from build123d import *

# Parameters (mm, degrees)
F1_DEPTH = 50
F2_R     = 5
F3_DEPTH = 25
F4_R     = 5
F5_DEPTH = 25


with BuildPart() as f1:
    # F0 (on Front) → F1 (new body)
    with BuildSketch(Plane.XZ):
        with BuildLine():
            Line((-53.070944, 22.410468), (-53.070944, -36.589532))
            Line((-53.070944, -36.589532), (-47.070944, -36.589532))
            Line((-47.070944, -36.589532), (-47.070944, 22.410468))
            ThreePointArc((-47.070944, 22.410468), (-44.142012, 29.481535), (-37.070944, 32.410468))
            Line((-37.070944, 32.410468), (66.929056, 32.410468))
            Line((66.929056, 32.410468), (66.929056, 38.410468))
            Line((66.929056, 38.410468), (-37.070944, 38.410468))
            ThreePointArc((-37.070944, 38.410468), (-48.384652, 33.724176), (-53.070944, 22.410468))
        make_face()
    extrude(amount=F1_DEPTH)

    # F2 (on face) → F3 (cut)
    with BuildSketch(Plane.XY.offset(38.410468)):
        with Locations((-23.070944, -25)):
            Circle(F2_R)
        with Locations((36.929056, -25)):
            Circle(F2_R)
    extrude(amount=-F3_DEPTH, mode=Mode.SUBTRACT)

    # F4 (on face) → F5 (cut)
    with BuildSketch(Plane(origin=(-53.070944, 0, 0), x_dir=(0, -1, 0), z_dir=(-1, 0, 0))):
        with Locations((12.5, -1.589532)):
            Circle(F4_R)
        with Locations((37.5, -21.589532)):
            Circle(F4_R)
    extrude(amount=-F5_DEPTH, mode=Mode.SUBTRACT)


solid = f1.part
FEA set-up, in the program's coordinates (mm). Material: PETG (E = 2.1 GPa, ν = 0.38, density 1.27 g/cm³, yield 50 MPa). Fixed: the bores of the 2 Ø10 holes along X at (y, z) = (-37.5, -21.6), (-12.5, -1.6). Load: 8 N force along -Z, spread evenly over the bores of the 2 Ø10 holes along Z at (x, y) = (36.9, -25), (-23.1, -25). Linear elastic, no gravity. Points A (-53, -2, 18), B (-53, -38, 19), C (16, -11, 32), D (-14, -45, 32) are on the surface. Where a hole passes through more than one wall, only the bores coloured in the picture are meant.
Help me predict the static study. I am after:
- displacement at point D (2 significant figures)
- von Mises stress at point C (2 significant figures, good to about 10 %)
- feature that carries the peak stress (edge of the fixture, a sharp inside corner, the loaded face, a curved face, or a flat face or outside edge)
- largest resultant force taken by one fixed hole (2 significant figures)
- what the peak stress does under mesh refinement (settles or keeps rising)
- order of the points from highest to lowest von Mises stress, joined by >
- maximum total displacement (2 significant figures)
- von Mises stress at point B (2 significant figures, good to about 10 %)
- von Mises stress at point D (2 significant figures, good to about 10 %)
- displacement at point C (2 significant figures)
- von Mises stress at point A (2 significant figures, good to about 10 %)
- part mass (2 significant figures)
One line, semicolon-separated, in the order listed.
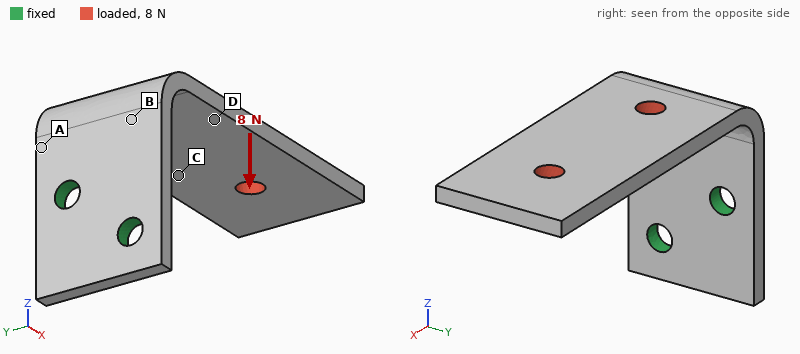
0.39 mm; 0.30 MPa; edge of the fixture; 7.8 N; keeps rising; A > B > D > C; 1.6 mm; 1.2 MPa; 0.74 MPa; 0.79 mm; 1.7 MPa; 67 g
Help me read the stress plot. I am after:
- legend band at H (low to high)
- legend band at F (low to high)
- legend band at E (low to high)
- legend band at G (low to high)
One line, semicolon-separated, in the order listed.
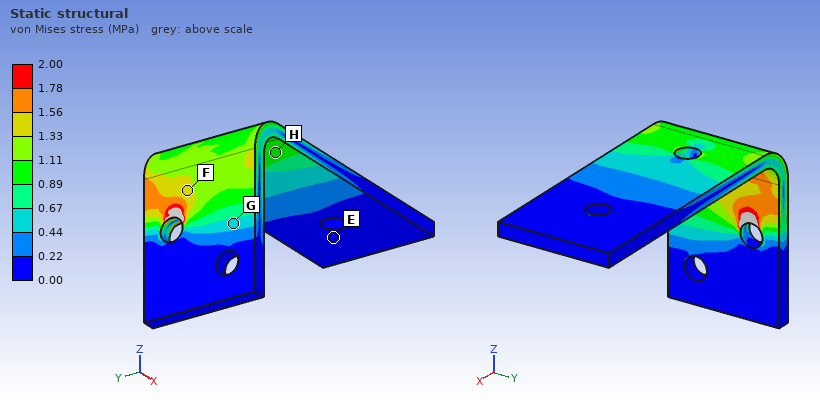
0.89 to 1.11 MPa; 1.33 to 1.56 MPa; 0.00 to 0.22 MPa; 0.44 to 0.67 MPa
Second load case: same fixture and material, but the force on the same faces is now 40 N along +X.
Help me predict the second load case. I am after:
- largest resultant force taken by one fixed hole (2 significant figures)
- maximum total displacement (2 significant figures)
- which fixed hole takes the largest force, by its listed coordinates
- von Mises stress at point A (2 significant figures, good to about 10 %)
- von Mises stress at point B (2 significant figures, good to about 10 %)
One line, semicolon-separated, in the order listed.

48 N; 1.8 mm; (-12.5, -1.6); 2.9 MPa; 1.6 MPa
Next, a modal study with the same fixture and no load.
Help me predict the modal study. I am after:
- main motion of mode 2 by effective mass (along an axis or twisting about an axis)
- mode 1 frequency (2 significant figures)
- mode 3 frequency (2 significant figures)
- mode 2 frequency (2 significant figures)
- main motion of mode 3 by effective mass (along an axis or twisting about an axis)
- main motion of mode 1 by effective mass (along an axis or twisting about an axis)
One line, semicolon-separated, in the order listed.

along Y; 64 Hz; 310 Hz; 110 Hz; along X; along Z
